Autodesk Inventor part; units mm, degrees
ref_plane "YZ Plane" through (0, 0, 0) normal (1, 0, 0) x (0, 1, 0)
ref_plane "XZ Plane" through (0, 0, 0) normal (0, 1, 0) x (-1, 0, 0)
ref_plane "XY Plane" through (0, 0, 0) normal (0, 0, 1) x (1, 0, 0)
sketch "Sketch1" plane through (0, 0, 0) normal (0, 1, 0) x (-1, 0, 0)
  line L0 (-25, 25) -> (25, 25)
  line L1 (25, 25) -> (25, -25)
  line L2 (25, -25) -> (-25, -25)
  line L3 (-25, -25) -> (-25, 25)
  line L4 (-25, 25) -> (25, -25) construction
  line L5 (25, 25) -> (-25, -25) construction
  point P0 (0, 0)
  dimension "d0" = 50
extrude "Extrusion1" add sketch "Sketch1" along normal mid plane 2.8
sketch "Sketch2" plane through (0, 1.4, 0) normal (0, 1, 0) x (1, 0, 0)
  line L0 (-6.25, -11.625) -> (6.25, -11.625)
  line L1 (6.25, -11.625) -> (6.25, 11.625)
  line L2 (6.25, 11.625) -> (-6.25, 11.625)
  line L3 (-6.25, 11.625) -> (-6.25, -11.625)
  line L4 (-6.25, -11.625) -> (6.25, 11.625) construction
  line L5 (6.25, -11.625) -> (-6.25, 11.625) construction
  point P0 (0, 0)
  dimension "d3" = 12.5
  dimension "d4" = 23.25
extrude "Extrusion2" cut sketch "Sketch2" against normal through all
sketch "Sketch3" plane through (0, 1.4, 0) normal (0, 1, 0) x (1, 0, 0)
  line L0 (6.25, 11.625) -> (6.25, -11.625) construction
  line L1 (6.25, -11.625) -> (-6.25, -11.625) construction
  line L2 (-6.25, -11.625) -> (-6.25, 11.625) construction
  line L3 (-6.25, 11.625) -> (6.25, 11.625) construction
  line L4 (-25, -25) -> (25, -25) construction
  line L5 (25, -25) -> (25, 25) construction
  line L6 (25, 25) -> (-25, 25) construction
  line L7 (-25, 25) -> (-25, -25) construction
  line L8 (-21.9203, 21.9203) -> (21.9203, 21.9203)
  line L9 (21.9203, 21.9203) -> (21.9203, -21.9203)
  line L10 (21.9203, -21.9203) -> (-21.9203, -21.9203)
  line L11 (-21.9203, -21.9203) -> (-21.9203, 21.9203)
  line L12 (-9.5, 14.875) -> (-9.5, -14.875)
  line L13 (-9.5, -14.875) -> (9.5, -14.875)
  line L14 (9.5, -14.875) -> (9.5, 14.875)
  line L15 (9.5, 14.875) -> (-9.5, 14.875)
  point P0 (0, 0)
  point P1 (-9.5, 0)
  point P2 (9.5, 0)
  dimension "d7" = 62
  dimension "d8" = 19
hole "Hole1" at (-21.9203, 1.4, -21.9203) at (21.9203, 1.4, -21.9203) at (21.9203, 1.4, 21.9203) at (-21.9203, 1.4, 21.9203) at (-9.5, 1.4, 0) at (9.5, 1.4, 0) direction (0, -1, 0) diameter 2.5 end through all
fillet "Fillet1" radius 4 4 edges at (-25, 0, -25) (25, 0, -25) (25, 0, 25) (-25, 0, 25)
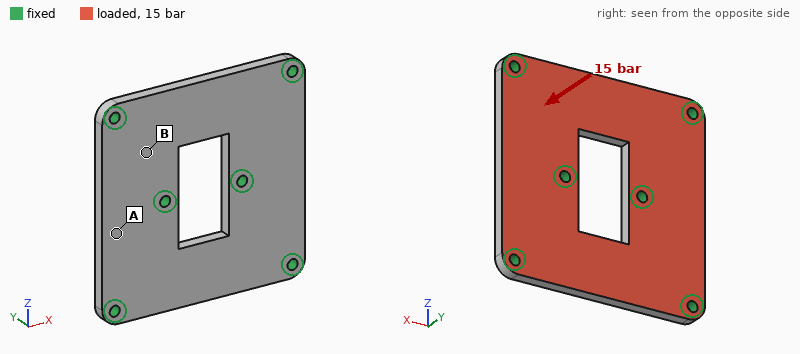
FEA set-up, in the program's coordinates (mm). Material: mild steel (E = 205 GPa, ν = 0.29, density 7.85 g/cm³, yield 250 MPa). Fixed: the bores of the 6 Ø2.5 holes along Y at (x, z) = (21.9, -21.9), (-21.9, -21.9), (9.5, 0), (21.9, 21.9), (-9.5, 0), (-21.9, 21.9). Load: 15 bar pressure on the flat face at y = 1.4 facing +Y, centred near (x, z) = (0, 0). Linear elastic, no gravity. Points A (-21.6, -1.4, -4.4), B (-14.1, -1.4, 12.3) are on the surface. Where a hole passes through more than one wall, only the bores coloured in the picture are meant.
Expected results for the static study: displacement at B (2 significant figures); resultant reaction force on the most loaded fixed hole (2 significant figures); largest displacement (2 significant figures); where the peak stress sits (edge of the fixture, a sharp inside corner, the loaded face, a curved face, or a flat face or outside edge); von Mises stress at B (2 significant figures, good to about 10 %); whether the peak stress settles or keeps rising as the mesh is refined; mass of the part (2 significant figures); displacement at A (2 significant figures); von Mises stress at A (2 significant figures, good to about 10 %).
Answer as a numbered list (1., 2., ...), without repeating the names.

1. 9.6 µm
2. 720 N
3. 32 µm
4. edge of the fixture
5. 60 MPa
6. keeps rising
7. 48 g
8. 7.9 µm
9. 26 MPa
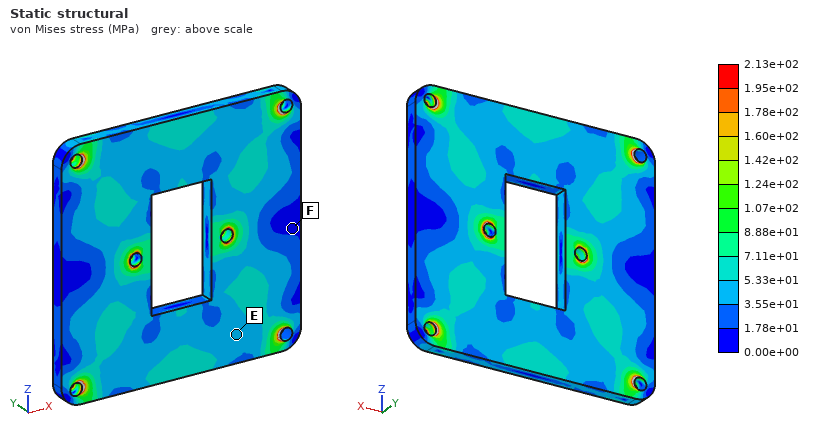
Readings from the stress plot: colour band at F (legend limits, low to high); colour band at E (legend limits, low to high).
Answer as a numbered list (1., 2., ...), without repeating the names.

1. 0.00e+00 to 1.78e+01 MPa
2. 3.55e+01 to 5.33e+01 MPa
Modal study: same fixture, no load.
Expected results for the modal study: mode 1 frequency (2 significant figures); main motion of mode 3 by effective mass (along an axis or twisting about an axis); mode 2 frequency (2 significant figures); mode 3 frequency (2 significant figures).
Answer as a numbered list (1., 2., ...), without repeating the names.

1. 8800 Hz
2. twisting about Z
3. 9100 Hz
4. 13 kHz
